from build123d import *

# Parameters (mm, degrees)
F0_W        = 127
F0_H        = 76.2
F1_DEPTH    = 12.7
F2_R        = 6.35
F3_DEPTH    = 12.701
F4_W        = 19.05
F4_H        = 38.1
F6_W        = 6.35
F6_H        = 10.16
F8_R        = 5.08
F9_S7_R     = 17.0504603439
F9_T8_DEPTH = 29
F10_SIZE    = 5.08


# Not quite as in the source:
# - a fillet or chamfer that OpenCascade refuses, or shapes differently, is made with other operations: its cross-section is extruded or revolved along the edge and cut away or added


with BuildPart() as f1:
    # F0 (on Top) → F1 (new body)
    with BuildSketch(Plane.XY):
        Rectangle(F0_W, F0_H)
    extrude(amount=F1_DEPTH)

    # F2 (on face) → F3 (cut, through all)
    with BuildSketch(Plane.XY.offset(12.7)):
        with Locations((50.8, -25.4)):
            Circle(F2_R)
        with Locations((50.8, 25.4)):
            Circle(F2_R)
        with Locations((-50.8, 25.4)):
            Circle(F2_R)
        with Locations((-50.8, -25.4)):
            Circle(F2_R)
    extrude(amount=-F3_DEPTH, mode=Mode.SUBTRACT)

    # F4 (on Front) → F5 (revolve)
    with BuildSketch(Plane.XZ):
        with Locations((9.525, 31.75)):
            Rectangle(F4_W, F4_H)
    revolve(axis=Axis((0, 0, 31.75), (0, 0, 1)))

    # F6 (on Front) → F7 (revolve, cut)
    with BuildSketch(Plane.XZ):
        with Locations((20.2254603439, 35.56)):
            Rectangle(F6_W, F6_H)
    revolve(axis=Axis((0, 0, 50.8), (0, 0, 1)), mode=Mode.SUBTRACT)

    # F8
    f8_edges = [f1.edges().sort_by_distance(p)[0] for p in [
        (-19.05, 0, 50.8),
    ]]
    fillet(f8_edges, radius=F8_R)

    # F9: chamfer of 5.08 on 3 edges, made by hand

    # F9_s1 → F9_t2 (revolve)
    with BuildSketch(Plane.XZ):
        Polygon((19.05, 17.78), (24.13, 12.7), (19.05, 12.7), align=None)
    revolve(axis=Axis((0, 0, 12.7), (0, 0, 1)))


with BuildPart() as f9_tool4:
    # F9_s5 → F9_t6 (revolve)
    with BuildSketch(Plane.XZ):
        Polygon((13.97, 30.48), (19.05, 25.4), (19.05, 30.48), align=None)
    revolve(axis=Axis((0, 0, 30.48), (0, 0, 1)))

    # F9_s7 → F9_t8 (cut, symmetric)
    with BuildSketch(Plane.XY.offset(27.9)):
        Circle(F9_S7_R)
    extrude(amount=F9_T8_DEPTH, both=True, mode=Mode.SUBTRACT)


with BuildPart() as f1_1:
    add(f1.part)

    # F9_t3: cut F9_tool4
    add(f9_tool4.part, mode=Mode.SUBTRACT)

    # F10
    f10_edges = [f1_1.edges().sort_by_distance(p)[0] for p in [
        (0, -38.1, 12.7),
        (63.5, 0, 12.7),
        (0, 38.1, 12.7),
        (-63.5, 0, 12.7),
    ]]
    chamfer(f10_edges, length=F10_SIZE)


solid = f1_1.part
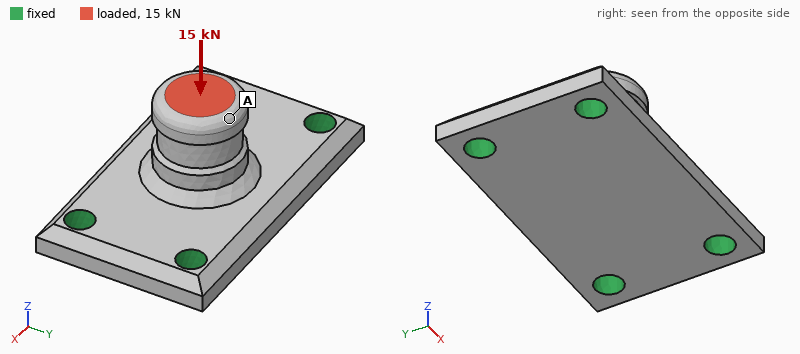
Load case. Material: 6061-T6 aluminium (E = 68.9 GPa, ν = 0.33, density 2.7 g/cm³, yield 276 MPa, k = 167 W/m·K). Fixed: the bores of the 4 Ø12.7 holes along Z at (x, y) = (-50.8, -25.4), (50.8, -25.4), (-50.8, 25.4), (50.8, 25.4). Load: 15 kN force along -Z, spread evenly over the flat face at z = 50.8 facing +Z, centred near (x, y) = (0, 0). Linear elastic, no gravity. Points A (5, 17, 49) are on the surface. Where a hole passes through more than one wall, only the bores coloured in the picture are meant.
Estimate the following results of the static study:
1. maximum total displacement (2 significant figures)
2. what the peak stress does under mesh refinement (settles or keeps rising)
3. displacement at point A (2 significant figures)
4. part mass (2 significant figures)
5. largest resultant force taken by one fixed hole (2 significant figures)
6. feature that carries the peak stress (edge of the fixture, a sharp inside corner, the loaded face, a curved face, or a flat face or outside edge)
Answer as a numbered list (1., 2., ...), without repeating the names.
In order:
1. 64 µm
2. keeps rising
3. 60 µm
4. 410 g
5. 4.0 kN
6. edge of the fixture
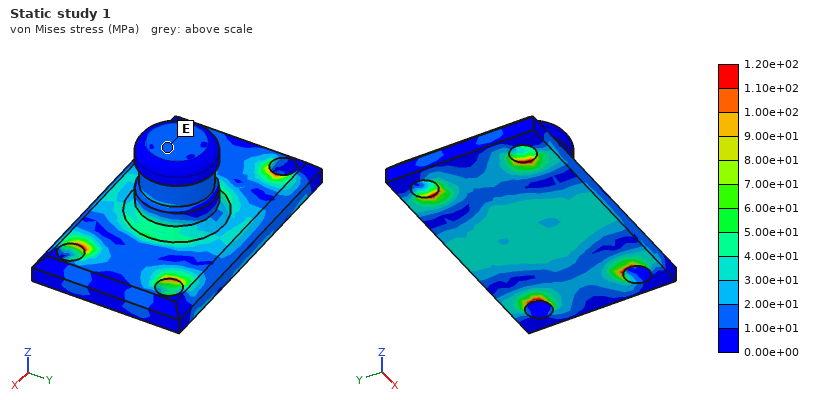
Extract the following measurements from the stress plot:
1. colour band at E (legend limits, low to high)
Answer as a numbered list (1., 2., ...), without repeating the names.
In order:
1. 1.00e+01 to 2.00e+01 MPa
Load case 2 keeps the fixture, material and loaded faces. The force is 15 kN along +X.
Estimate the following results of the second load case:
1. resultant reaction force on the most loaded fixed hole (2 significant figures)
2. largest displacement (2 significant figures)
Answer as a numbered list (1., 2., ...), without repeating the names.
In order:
1. 6.1 kN
2. 0.16 mm
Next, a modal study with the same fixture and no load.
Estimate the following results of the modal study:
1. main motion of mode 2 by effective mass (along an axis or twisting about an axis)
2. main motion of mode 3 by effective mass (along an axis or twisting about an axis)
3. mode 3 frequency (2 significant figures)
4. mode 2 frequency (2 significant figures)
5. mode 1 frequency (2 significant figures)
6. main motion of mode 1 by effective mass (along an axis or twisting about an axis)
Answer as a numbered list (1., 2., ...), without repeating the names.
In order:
1. along Z
2. along X
3. 7500 Hz
4. 5300 Hz
5. 5100 Hz
6. along Y
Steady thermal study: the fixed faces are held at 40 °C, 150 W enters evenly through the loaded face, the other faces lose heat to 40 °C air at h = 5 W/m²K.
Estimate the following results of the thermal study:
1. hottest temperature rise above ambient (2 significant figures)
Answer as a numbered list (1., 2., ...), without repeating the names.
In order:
1. 58 K
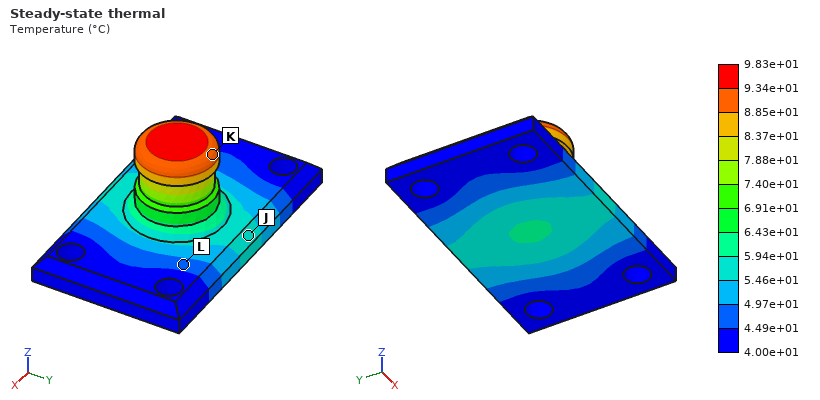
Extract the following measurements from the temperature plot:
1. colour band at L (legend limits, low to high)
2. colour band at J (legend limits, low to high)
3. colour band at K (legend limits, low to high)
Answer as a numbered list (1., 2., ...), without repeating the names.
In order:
1. 4.49e+01 to 4.97e+01 °C
2. 5.46e+01 to 5.94e+01 °C
3. 8.85e+01 to 9.34e+01 °C
